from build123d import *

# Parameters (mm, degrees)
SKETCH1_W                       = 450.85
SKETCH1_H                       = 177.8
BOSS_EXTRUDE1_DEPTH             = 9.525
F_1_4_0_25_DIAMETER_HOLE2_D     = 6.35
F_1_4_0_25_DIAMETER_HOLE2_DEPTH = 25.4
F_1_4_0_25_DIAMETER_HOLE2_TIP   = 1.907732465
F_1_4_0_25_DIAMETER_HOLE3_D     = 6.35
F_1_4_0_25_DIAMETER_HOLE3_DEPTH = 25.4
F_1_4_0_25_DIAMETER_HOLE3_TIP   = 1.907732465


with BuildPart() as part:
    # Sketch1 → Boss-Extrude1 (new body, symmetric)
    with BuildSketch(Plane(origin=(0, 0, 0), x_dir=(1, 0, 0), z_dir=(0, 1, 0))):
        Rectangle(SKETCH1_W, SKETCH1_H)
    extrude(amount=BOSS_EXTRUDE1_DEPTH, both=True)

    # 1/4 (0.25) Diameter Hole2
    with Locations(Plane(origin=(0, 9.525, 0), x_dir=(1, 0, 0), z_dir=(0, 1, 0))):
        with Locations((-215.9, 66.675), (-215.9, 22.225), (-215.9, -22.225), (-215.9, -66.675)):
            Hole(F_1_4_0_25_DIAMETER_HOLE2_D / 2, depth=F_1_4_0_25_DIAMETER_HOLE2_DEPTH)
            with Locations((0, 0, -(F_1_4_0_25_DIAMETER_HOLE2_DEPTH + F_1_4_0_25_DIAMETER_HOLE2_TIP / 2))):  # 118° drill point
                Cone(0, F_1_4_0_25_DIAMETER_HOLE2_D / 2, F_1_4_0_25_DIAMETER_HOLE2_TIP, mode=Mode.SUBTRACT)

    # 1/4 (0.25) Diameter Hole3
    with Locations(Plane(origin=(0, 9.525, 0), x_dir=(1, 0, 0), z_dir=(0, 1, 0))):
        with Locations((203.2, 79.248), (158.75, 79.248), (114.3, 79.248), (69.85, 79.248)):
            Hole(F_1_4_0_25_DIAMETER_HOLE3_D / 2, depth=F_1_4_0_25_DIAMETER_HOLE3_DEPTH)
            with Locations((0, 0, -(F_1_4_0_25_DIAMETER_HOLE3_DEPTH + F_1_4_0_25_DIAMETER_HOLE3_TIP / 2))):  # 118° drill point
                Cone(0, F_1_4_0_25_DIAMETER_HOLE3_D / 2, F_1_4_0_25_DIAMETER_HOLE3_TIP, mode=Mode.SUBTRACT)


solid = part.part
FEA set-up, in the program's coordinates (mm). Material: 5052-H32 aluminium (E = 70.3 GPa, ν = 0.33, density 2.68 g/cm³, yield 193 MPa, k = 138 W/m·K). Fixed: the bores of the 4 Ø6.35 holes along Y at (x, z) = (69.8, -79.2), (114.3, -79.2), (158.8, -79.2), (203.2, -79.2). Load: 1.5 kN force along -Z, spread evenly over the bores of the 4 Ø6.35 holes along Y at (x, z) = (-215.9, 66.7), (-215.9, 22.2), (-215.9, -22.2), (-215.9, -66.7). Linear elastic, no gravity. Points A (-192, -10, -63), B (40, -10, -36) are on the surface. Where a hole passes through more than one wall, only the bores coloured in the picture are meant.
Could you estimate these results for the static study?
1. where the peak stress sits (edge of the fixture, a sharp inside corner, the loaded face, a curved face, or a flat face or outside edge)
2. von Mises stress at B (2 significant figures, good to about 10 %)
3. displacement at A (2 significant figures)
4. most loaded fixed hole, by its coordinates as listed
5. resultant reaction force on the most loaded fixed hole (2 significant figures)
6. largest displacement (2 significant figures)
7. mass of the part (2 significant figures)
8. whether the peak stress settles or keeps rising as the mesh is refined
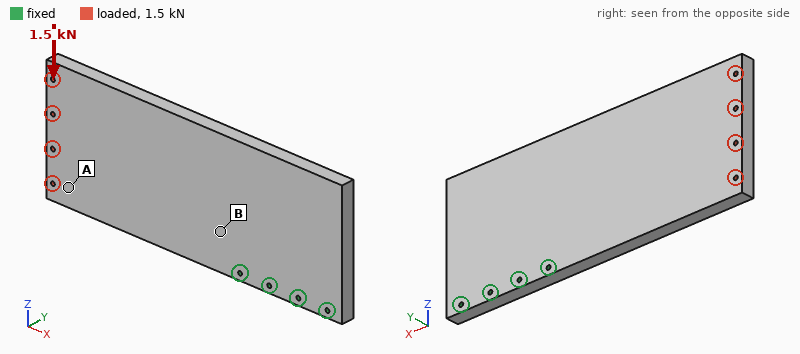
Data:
edge of the fixture
2.2 MPa
52 µm
(69.8, -79.2)
4.7 kN
65 µm
4.1 kg
keeps rising
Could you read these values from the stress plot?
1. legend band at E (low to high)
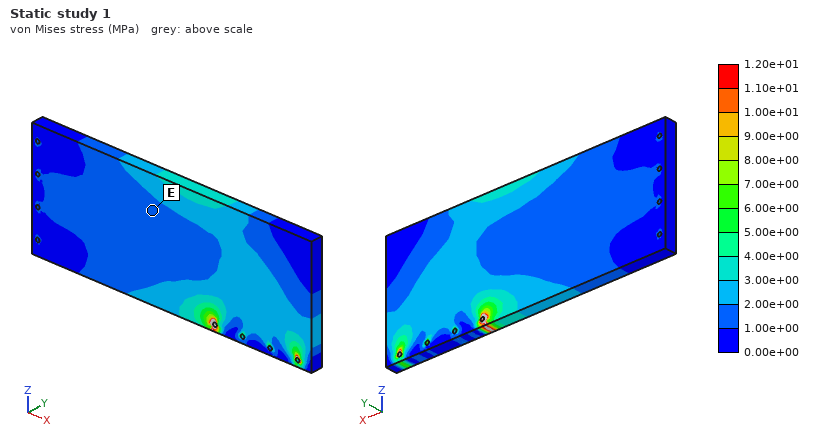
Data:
1.00e+00 to 2.00e+00 MPa
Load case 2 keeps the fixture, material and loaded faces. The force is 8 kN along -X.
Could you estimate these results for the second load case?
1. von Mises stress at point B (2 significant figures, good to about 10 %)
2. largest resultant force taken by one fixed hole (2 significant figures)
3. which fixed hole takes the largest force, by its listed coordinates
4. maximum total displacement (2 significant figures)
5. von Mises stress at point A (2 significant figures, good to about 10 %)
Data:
2.7 MPa
5.3 kN
(69.8, -79.2)
53 µm
2.9 MPa
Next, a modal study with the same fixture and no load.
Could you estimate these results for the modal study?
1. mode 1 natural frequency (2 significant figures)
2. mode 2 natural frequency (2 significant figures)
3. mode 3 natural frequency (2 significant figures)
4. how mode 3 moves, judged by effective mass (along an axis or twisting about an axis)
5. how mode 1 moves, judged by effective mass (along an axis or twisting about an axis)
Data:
140 Hz
370 Hz
710 Hz
along Y
along Y
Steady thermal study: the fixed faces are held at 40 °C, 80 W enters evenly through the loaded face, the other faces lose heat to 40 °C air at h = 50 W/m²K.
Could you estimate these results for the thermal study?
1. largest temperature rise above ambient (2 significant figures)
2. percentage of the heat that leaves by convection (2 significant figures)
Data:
25 K
84 %
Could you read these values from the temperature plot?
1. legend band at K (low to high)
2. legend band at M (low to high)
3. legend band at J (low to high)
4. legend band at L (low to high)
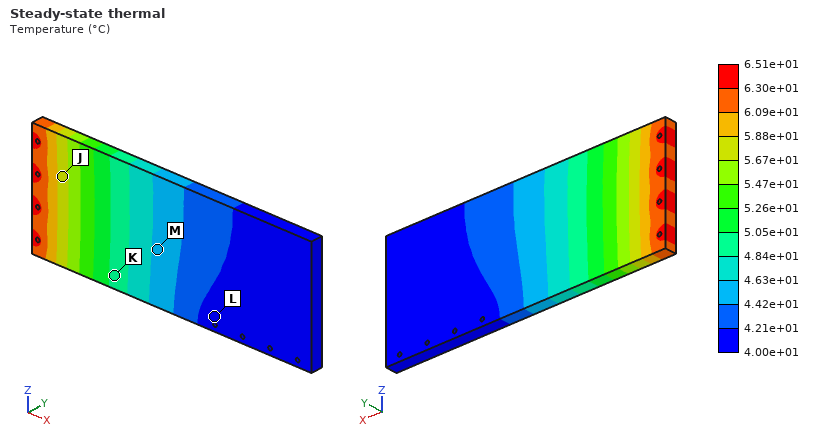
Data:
4.84e+01 to 5.05e+01 °C
4.42e+01 to 4.63e+01 °C
5.67e+01 to 5.88e+01 °C
4.00e+01 to 4.21e+01 °C
